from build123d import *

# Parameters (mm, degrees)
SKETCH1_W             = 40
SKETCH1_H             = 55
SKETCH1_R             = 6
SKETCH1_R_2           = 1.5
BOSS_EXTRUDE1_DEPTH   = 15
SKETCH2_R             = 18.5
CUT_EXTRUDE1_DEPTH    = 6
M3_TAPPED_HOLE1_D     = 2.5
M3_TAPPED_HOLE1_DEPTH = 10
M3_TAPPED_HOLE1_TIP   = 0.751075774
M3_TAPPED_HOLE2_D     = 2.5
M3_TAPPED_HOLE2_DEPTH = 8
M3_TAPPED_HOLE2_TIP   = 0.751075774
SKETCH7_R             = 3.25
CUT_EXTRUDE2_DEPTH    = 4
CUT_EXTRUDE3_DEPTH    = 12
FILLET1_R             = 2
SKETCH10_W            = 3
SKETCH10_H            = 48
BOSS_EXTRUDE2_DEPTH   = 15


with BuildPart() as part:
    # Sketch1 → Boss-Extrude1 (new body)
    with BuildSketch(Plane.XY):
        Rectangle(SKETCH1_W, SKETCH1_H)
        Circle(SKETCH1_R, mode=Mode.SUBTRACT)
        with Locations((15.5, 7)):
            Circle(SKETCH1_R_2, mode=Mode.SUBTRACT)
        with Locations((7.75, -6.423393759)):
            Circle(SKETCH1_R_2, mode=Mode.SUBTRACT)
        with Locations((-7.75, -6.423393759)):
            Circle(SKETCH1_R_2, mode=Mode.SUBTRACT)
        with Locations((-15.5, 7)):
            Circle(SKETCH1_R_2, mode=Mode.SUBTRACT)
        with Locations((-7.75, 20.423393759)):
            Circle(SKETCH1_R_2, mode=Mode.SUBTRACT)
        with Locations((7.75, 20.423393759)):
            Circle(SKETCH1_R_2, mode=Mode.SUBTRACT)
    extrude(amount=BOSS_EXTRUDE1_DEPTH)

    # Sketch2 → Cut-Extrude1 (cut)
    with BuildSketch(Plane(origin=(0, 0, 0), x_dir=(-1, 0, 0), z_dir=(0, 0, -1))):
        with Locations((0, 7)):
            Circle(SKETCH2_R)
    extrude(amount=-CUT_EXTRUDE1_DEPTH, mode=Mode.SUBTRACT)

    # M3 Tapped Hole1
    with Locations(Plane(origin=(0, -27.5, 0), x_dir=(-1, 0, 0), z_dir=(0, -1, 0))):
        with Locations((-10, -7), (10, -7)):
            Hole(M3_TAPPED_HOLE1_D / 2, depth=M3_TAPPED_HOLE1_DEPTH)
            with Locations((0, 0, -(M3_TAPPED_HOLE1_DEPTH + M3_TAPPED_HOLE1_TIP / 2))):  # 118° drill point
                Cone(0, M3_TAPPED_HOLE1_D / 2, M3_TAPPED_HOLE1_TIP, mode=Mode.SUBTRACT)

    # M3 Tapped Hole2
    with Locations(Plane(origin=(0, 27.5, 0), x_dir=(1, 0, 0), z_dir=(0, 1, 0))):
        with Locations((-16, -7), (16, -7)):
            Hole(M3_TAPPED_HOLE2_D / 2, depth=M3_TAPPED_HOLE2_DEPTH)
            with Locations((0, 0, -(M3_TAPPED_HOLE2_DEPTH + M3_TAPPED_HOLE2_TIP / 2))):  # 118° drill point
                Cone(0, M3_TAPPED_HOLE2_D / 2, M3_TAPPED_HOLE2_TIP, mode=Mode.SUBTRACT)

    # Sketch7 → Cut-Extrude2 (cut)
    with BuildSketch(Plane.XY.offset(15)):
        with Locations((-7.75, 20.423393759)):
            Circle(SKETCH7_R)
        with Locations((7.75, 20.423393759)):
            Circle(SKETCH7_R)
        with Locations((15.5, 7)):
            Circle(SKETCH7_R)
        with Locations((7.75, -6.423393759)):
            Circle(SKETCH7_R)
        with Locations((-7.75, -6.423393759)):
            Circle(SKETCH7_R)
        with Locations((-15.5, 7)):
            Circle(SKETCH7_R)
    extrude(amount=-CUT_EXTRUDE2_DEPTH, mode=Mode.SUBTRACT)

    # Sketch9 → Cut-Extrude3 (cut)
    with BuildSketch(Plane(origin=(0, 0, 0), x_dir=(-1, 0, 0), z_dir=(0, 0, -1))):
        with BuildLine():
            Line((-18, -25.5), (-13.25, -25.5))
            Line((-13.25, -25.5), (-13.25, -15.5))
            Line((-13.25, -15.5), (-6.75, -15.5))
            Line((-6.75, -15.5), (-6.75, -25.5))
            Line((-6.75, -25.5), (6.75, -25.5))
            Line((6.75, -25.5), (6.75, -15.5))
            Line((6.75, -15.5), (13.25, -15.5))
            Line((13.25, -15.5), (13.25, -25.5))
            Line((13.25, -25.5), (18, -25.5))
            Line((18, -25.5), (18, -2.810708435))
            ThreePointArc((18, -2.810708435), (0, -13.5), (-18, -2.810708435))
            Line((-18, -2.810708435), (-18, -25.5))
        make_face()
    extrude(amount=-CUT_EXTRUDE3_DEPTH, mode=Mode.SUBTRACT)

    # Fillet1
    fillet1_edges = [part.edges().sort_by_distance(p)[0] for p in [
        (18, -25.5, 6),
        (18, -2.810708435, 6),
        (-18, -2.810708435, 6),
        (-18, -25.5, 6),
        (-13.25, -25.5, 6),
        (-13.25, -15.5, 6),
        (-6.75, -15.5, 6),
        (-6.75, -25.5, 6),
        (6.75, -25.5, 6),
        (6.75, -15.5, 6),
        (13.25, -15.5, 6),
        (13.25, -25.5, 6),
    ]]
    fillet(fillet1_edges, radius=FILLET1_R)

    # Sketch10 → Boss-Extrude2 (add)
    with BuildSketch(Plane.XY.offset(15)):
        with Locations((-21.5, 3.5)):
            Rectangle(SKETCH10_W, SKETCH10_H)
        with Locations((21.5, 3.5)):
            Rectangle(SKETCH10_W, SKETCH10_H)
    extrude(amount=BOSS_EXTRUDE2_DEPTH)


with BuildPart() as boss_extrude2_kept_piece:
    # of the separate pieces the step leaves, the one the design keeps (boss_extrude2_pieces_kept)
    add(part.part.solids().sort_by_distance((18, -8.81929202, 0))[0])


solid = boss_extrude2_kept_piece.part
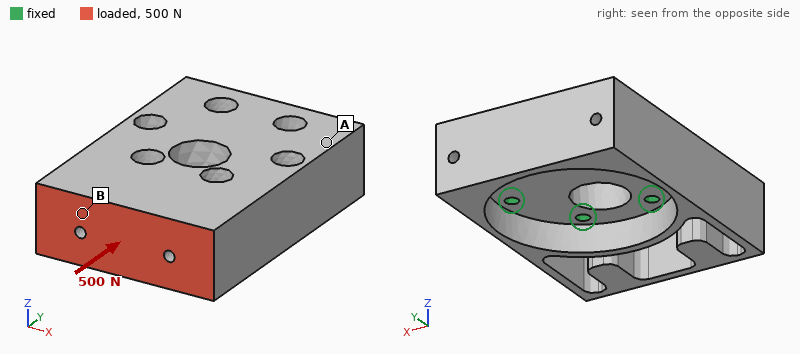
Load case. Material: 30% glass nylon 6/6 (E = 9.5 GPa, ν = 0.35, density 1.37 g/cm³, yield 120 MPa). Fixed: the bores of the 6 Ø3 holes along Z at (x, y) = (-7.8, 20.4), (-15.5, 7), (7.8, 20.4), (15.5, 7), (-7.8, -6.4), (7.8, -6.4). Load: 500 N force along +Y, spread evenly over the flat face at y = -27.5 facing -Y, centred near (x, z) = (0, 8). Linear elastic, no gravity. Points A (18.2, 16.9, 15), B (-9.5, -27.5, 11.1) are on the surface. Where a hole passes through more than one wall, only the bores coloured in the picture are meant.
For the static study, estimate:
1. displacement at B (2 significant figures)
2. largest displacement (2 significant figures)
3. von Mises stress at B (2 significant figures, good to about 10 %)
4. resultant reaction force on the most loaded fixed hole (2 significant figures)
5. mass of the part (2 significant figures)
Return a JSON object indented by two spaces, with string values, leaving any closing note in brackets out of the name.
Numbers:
{
  "displacement at B": "0.060 mm",
  "largest displacement": "0.12 mm",
  "von Mises stress at B": "5.5 MPa",
  "resultant reaction force on the most loaded fixed hole": "120 N",
  "mass of the part": "27 g"
}
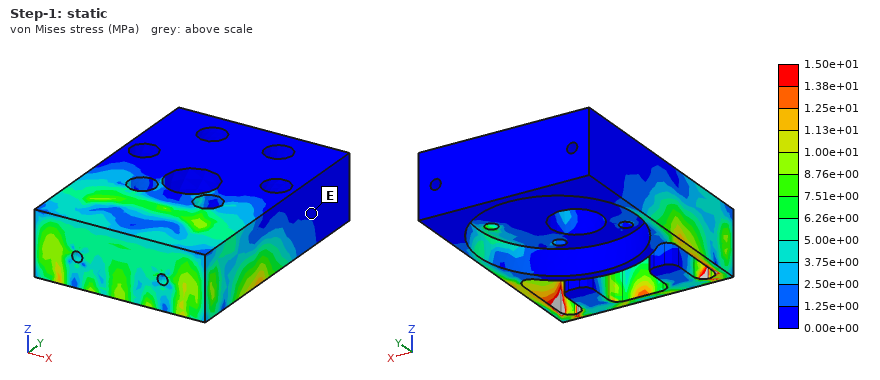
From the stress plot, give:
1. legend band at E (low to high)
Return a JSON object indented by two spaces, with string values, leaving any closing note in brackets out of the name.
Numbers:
{
  "legend band at E": "0.00e+00 to 1.25e+00 MPa"
}
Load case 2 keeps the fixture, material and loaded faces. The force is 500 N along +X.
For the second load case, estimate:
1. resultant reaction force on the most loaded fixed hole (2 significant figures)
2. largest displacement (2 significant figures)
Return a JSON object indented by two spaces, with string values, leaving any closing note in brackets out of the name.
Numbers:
{
  "resultant reaction force on the most loaded fixed hole": "370 N",
  "largest displacement": "0.15 mm"
}
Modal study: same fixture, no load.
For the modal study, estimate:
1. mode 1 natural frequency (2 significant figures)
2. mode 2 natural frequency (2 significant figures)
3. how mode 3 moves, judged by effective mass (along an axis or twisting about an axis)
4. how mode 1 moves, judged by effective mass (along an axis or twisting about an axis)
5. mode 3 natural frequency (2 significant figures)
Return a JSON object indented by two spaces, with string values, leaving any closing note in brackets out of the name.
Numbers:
{
  "mode 1 natural frequency": "3700 Hz",
  "mode 2 natural frequency": "4200 Hz",
  "how mode 3 moves, judged by effective mass": "along X",
  "how mode 1 moves, judged by effective mass": "along Z",
  "mode 3 natural frequency": "8900 Hz"
}
